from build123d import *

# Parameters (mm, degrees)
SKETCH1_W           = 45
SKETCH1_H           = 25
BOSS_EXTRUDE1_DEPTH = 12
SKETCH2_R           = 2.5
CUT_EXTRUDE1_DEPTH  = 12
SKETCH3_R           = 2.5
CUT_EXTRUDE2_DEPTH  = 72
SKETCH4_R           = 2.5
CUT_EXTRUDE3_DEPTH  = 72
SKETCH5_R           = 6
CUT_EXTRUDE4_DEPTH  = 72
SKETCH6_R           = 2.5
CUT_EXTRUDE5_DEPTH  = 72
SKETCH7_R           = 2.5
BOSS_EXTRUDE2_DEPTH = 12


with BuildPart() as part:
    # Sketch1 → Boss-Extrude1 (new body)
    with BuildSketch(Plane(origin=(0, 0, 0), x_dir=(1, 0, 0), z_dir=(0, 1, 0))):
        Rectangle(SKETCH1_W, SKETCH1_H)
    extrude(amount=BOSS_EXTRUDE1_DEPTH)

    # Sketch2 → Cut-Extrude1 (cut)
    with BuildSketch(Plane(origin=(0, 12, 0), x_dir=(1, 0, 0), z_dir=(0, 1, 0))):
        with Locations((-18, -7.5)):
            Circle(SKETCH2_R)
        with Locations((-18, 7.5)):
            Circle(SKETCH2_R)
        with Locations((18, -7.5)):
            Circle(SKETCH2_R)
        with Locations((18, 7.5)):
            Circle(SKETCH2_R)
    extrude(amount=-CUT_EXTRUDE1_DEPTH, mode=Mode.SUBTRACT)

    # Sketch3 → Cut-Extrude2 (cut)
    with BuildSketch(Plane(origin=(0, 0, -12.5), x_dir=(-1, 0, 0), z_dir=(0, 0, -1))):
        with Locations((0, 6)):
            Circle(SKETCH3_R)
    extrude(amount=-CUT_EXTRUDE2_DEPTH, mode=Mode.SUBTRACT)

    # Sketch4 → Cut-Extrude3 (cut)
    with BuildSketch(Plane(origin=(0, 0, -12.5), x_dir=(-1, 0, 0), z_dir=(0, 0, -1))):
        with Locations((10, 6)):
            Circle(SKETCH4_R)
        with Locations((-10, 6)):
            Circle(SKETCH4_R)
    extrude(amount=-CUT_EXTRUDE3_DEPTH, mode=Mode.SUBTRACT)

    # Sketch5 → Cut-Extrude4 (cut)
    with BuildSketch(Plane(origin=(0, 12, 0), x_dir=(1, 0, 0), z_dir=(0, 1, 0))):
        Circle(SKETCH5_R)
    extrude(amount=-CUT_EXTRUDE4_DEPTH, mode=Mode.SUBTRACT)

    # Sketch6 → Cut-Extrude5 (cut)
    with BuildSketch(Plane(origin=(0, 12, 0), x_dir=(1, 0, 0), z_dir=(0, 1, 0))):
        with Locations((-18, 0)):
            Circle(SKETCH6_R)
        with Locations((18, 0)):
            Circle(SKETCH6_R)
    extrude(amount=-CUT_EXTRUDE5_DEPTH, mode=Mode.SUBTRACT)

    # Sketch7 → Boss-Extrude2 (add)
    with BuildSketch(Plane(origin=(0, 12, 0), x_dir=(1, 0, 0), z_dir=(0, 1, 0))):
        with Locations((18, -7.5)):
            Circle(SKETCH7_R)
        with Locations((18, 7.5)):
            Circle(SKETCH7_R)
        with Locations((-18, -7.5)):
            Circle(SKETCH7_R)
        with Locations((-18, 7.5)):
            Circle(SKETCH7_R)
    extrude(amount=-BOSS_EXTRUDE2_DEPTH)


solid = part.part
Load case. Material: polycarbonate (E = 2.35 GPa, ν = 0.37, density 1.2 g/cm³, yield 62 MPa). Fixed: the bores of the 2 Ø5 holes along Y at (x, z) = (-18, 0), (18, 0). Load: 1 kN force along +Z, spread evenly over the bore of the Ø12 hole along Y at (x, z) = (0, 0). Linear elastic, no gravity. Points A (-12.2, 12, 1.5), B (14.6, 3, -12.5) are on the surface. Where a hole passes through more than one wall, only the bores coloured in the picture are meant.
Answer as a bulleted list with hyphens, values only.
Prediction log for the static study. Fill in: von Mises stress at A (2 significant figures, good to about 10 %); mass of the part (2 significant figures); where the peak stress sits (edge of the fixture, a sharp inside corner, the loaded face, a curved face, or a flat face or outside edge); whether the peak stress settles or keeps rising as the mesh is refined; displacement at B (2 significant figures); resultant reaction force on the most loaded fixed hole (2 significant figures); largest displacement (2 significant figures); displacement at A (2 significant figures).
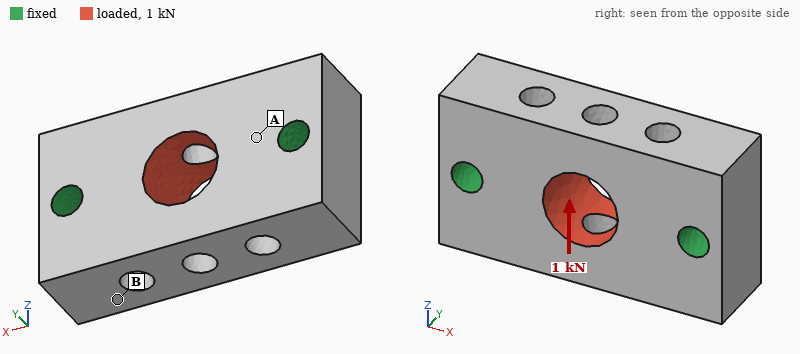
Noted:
- 5.9 MPa
- 13 g
- edge of the fixture
- keeps rising
- 31 µm
- 500 N
- 71 µm
- 24 µm
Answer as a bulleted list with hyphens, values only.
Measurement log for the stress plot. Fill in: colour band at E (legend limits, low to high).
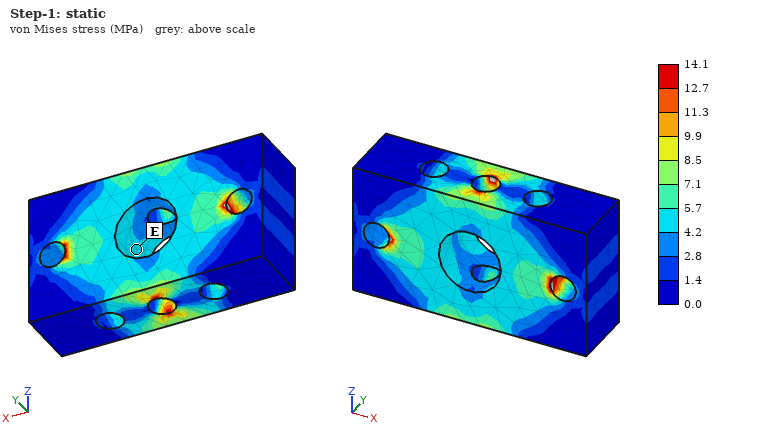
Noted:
- 4.2 to 5.7 MPa
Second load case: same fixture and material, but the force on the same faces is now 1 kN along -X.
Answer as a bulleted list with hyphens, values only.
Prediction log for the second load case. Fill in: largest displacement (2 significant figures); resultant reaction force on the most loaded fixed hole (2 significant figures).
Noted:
- 29 µm
- 500 N
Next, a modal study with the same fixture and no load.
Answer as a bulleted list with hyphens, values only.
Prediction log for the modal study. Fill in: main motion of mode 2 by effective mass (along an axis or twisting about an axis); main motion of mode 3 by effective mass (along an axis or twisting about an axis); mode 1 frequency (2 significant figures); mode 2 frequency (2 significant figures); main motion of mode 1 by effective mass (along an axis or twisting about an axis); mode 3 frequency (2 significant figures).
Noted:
- twisting about X
- along Z
- 7200 Hz
- 7600 Hz
- along Y
- 9100 Hz
